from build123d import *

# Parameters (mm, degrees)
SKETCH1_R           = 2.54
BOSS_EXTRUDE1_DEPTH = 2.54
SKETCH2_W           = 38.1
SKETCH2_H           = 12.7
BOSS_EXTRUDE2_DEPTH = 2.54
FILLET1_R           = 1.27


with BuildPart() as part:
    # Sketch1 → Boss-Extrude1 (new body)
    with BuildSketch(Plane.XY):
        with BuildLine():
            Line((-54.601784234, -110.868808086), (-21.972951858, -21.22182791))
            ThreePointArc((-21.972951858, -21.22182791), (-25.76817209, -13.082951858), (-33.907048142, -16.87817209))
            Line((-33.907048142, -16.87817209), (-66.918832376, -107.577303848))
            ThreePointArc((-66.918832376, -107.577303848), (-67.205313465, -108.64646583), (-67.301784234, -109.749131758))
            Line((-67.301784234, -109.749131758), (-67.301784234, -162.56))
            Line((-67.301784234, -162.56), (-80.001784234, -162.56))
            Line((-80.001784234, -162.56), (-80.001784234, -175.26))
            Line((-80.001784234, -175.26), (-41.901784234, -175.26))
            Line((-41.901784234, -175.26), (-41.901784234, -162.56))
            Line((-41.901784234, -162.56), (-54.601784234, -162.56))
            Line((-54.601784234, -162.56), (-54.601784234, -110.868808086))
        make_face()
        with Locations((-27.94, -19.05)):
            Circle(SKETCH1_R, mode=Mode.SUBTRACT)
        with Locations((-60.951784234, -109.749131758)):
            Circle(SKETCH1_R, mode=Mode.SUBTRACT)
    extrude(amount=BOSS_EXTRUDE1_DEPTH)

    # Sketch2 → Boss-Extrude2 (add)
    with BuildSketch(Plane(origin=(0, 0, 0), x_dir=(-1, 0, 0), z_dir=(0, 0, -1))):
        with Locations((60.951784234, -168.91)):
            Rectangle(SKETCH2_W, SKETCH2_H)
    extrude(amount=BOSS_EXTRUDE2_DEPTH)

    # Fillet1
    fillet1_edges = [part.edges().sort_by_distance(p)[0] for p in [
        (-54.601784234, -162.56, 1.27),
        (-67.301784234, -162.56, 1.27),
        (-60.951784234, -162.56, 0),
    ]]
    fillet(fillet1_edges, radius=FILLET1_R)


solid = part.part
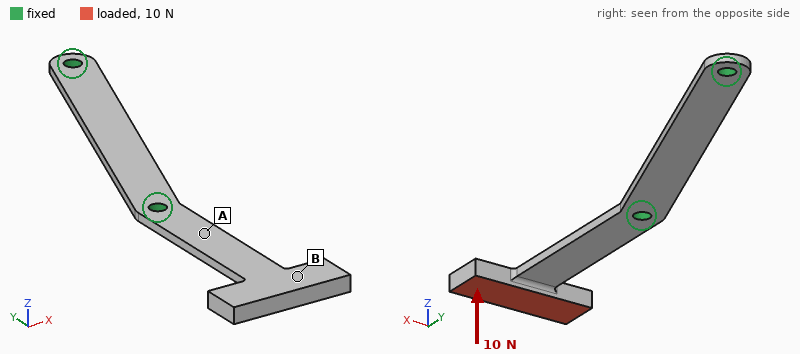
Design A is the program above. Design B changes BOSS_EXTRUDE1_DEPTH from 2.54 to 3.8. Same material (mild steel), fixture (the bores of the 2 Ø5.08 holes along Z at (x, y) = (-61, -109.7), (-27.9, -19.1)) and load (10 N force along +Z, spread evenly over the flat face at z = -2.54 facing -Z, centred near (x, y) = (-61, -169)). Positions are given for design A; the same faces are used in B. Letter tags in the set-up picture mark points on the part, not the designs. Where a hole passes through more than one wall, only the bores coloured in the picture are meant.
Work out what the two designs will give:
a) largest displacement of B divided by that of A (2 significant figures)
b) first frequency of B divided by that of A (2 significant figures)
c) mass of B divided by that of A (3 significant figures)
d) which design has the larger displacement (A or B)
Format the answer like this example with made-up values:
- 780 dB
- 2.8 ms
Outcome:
- 0.30
- 1.6
- 1.41
- A
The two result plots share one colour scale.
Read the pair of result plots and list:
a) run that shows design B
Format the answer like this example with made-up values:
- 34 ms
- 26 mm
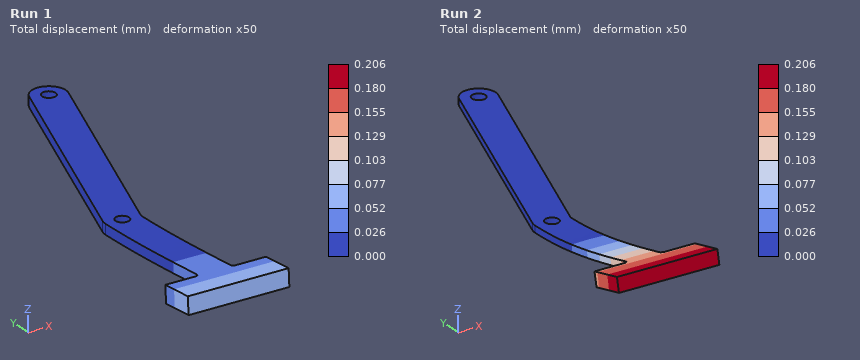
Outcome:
- Run 1
